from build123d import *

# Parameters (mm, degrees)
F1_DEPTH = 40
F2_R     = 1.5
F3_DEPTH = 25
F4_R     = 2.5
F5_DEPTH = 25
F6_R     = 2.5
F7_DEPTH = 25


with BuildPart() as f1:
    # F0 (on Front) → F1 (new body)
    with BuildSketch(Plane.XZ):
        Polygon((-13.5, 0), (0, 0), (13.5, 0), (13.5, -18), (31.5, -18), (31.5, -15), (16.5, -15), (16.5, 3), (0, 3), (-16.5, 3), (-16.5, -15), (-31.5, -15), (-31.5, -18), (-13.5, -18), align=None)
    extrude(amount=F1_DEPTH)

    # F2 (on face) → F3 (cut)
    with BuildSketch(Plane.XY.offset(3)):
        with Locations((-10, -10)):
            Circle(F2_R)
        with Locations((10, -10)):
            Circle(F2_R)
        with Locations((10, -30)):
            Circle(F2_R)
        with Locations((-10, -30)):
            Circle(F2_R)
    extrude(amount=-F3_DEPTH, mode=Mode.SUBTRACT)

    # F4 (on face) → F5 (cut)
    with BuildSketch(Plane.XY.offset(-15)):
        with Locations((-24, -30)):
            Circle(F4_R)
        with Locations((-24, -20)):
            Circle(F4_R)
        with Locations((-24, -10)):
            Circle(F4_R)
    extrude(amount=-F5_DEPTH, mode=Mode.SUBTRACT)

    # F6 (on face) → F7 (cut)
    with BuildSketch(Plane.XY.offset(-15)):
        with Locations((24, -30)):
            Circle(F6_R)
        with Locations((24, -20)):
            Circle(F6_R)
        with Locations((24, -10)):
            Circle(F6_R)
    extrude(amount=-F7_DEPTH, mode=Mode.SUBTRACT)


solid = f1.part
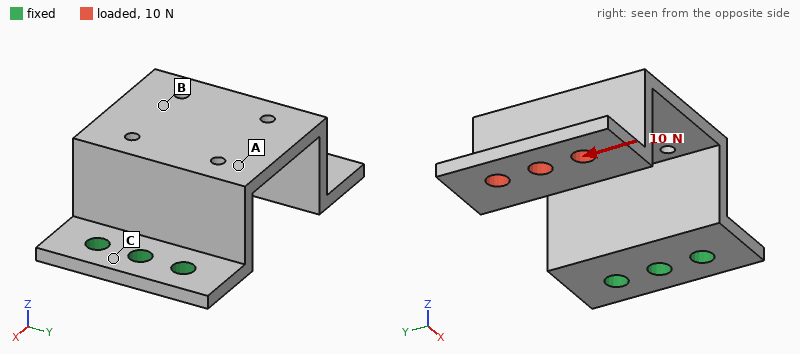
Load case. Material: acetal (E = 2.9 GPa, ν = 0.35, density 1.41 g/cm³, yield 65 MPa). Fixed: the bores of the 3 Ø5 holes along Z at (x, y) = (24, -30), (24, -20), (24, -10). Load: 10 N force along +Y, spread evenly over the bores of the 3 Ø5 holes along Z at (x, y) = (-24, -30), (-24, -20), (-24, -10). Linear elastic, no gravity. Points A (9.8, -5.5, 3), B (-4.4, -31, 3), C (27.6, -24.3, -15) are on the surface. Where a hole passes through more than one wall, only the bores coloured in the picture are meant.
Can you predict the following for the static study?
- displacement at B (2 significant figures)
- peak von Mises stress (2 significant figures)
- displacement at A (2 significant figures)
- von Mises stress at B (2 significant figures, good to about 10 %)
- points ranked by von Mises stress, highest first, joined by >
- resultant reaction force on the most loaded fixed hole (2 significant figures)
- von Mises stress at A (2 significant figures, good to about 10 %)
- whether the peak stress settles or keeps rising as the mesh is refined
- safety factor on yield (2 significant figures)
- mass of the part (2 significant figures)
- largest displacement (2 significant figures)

0.25 mm
5.4 MPa
0.19 mm
2.0 MPa
A > B > C
19 N
3.0 MPa
settles
12
16 g
0.86 mm
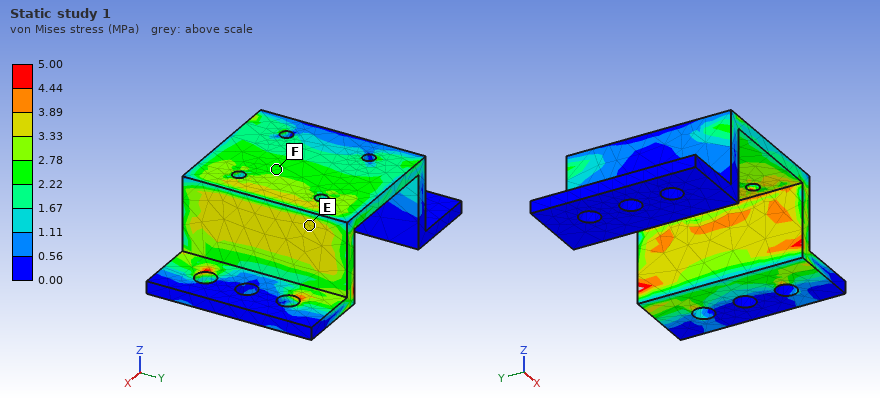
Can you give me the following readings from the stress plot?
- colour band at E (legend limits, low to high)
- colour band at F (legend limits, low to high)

3.33 to 3.89 MPa
2.22 to 2.78 MPa
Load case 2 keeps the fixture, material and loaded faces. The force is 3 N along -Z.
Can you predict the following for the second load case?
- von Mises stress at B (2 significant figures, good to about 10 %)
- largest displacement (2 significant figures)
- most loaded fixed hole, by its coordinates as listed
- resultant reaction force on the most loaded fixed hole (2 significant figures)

0.84 MPa
0.82 mm
(24, -20)
1.9 N
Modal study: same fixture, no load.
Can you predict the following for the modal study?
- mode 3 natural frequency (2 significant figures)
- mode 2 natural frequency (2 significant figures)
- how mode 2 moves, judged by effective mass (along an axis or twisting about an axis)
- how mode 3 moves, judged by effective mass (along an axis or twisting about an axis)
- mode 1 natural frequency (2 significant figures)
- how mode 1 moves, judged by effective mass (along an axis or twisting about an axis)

420 Hz
270 Hz
along Y
along X
150 Hz
along Z
